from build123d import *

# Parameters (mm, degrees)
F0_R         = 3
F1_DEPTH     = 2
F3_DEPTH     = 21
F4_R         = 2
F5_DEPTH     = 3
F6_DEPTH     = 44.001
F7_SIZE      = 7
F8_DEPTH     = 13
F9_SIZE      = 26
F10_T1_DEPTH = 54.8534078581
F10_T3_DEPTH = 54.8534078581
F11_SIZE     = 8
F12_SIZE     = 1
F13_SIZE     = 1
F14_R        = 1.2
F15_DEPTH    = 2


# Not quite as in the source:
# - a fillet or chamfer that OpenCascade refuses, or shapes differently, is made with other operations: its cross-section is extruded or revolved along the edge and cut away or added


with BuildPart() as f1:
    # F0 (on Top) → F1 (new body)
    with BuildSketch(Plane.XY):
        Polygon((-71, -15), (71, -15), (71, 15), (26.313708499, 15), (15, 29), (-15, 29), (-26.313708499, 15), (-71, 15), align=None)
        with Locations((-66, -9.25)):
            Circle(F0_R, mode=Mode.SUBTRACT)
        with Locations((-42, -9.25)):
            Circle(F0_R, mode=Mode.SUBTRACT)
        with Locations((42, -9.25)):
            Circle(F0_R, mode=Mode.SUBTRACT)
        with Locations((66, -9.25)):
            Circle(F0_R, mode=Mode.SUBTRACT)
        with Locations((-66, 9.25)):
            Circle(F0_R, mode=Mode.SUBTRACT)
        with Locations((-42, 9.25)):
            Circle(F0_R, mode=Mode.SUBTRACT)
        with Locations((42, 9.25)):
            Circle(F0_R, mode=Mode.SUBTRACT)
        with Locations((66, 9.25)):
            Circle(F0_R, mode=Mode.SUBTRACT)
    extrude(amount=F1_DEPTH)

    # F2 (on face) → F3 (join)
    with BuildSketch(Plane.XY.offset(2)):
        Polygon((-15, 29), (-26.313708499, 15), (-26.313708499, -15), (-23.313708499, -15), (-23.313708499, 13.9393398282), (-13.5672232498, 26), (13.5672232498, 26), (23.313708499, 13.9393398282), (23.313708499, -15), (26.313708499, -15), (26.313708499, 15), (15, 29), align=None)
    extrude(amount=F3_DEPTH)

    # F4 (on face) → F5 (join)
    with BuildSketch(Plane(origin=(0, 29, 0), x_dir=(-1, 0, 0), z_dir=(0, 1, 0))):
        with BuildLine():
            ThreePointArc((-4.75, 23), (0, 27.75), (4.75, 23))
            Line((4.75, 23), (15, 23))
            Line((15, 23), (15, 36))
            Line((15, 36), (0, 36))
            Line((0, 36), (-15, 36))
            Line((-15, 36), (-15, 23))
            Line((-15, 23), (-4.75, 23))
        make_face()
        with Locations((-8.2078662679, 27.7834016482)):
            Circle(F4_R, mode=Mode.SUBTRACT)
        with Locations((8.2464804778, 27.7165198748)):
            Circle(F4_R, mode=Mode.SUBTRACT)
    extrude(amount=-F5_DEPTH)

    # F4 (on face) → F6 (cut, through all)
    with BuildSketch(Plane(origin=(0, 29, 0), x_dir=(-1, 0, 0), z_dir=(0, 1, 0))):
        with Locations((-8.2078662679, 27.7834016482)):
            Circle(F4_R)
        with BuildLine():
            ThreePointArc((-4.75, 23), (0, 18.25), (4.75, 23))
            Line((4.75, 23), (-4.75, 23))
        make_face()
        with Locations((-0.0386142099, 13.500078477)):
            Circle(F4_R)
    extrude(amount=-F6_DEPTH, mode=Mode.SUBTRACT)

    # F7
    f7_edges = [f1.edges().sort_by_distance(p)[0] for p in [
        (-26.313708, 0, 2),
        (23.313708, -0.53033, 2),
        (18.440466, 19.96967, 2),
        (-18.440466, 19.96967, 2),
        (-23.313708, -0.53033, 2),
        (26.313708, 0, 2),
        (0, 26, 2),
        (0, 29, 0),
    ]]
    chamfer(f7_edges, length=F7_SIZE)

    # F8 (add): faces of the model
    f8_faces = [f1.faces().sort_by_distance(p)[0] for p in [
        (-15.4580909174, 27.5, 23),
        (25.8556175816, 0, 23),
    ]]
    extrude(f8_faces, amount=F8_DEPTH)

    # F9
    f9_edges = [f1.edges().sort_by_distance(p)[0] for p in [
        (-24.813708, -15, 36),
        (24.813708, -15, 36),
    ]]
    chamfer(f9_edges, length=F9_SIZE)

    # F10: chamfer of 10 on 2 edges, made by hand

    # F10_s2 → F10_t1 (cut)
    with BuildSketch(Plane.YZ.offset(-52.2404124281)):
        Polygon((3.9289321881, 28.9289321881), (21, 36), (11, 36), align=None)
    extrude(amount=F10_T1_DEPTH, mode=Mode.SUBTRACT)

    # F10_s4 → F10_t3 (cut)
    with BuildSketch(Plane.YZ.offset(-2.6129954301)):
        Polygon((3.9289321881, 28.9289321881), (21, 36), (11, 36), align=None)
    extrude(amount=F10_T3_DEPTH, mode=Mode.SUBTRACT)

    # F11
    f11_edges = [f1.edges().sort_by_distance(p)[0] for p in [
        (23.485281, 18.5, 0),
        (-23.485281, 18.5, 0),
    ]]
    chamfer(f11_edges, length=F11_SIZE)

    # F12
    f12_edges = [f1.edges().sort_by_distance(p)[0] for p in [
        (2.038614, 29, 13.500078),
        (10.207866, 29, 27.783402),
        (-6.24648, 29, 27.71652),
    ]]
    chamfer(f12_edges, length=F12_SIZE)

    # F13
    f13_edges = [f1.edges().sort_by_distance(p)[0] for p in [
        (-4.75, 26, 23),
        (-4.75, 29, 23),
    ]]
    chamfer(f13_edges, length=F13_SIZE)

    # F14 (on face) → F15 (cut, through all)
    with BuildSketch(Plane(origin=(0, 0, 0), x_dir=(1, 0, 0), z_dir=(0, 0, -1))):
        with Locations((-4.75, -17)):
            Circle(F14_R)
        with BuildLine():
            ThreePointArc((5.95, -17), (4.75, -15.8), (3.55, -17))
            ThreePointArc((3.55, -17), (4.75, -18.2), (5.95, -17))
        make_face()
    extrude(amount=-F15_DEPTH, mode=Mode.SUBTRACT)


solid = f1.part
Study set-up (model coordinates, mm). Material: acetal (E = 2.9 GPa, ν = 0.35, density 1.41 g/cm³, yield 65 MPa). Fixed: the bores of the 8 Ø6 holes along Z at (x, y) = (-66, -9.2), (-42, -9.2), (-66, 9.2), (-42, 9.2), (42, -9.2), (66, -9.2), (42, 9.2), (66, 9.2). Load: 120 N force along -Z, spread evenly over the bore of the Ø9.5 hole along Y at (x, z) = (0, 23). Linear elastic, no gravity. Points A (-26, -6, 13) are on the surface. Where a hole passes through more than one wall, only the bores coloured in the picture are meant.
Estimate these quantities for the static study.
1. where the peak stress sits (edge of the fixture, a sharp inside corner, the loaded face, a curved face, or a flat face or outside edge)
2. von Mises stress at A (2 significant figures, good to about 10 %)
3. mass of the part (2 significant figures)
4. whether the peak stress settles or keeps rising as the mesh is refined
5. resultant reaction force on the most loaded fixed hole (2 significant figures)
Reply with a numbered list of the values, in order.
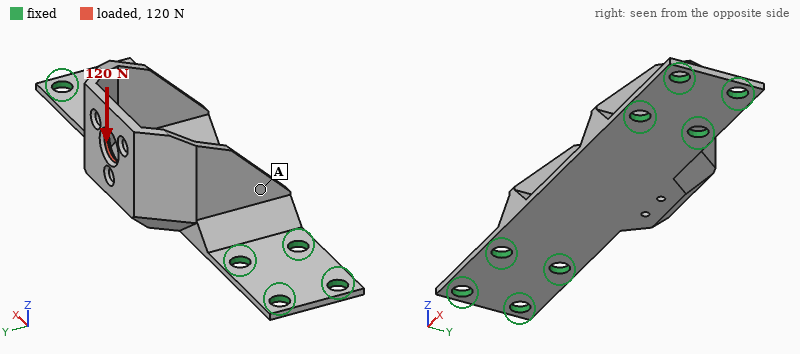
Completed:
1. edge of the fixture
2. 4.5 MPa
3. 30 g
4. keeps rising
5. 150 N
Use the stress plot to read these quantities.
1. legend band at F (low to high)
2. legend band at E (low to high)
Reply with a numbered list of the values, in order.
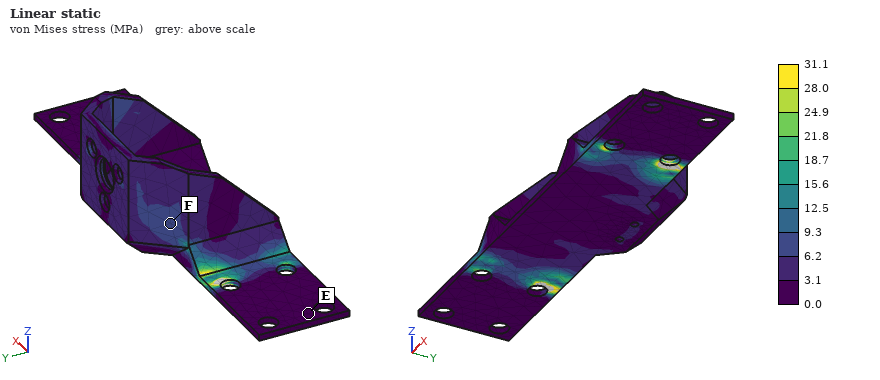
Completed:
1. 6.2 to 9.3 MPa
2. 0.0 to 3.1 MPa
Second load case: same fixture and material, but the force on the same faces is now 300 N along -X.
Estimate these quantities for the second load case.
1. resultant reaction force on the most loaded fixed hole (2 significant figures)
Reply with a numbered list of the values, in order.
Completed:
1. 150 N
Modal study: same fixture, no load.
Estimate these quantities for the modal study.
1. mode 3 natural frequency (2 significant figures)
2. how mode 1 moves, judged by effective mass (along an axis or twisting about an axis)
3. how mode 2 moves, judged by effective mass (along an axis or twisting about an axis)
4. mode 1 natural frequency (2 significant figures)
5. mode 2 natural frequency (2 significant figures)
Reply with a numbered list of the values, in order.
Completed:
1. 950 Hz
2. along Z
3. along Z
4. 520 Hz
5. 820 Hz
